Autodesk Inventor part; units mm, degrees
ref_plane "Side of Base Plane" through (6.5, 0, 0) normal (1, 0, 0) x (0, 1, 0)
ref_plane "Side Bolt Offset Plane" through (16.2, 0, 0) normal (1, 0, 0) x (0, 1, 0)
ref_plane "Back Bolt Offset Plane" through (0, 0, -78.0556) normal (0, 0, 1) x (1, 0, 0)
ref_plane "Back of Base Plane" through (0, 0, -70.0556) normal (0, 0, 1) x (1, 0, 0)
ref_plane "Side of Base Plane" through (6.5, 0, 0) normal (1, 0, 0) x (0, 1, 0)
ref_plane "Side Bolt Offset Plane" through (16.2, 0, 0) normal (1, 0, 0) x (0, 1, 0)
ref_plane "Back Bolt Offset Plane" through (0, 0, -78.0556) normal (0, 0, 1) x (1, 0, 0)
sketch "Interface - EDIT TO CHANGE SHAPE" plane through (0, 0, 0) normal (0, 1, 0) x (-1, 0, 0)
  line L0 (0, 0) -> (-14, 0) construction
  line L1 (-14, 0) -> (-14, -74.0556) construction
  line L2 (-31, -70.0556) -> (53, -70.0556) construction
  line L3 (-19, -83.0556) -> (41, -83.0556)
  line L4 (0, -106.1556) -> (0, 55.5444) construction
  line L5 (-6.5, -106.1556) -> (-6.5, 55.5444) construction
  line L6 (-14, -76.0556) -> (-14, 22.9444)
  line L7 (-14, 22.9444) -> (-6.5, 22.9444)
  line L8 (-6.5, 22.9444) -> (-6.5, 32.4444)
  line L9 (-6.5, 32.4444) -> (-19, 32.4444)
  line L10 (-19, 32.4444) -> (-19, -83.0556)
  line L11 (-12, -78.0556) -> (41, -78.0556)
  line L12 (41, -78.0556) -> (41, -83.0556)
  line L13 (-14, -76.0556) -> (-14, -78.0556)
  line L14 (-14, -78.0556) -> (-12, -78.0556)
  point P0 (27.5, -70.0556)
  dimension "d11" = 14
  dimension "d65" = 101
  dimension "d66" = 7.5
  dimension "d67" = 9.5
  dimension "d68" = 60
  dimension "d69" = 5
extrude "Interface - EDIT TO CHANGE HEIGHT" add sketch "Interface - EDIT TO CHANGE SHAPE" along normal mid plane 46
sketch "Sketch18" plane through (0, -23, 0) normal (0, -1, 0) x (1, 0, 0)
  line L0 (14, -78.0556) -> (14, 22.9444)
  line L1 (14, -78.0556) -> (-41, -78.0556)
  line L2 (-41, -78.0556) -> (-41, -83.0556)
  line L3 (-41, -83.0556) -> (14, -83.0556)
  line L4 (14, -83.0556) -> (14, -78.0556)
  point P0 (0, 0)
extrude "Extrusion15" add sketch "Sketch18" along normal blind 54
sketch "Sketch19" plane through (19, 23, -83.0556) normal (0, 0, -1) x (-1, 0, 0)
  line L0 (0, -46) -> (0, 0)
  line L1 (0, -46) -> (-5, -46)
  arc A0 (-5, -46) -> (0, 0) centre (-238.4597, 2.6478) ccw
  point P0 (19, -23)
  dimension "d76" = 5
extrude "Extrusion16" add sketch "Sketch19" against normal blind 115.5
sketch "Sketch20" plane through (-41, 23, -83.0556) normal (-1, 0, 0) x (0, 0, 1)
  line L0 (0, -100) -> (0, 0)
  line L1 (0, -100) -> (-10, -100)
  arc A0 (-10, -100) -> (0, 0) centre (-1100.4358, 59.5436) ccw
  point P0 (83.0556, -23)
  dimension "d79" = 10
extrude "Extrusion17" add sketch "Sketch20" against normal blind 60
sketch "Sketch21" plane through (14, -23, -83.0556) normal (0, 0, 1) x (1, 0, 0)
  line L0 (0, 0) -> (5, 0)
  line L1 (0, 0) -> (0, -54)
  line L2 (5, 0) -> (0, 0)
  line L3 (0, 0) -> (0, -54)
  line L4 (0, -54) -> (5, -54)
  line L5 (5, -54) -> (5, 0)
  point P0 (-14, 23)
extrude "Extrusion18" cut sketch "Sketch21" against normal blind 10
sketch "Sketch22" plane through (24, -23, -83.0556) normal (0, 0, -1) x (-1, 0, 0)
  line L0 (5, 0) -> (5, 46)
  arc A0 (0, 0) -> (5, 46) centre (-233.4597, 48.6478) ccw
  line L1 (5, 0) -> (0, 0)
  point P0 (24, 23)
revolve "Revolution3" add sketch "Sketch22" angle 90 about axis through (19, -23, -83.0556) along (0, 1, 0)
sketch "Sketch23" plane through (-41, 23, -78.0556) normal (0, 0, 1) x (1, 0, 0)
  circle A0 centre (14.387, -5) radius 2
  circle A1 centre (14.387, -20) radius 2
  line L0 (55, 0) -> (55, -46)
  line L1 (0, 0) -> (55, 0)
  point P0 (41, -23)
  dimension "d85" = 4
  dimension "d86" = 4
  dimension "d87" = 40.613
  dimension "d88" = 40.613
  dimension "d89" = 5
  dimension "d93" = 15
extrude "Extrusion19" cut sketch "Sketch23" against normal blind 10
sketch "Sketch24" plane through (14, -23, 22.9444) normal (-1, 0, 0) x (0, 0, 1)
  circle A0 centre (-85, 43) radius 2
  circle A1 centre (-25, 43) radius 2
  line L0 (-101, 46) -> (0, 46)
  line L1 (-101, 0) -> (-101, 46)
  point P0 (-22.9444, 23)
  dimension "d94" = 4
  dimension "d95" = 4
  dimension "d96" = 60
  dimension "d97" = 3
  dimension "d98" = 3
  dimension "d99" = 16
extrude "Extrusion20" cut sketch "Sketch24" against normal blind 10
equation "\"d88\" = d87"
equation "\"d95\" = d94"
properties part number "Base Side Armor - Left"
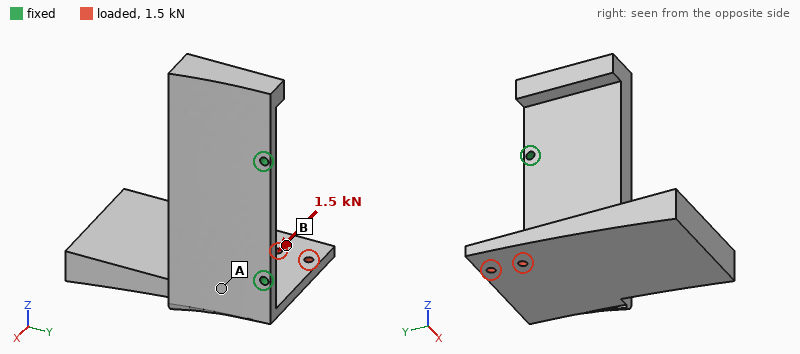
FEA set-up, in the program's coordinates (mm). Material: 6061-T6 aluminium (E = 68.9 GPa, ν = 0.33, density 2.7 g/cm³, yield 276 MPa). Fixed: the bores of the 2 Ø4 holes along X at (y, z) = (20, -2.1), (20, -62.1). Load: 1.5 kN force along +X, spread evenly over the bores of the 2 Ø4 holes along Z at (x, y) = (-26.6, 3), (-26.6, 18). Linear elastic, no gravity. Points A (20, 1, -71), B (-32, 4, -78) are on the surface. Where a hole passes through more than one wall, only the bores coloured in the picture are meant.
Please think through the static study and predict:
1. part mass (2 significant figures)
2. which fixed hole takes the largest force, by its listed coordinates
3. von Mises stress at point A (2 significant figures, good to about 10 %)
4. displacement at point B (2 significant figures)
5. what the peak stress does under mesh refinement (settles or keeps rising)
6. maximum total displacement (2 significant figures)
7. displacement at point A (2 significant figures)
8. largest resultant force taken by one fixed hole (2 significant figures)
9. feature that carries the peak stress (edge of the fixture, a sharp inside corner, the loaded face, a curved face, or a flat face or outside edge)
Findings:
240 g
(20, -62.1)
41 MPa
0.45 mm
keeps rising
0.77 mm
0.14 mm
1.8 kN
edge of the fixture
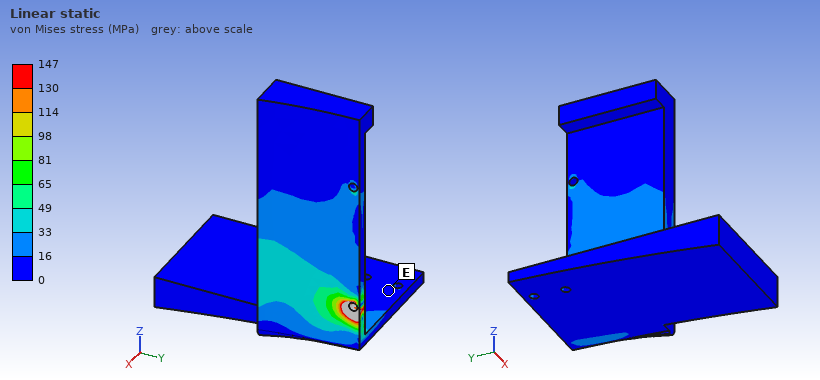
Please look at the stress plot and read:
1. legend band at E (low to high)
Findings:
0 to 16 MPa
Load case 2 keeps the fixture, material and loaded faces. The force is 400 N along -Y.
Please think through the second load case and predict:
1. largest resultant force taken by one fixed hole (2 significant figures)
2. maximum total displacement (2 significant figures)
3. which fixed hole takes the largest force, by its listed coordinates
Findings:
530 N
0.90 mm
(20, -62.1)
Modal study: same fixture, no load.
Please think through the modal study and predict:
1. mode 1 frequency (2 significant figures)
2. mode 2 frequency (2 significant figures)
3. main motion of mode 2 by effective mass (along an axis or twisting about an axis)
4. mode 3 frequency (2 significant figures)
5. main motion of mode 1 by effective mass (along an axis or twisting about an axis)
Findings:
280 Hz
500 Hz
along Z
1200 Hz
along X
